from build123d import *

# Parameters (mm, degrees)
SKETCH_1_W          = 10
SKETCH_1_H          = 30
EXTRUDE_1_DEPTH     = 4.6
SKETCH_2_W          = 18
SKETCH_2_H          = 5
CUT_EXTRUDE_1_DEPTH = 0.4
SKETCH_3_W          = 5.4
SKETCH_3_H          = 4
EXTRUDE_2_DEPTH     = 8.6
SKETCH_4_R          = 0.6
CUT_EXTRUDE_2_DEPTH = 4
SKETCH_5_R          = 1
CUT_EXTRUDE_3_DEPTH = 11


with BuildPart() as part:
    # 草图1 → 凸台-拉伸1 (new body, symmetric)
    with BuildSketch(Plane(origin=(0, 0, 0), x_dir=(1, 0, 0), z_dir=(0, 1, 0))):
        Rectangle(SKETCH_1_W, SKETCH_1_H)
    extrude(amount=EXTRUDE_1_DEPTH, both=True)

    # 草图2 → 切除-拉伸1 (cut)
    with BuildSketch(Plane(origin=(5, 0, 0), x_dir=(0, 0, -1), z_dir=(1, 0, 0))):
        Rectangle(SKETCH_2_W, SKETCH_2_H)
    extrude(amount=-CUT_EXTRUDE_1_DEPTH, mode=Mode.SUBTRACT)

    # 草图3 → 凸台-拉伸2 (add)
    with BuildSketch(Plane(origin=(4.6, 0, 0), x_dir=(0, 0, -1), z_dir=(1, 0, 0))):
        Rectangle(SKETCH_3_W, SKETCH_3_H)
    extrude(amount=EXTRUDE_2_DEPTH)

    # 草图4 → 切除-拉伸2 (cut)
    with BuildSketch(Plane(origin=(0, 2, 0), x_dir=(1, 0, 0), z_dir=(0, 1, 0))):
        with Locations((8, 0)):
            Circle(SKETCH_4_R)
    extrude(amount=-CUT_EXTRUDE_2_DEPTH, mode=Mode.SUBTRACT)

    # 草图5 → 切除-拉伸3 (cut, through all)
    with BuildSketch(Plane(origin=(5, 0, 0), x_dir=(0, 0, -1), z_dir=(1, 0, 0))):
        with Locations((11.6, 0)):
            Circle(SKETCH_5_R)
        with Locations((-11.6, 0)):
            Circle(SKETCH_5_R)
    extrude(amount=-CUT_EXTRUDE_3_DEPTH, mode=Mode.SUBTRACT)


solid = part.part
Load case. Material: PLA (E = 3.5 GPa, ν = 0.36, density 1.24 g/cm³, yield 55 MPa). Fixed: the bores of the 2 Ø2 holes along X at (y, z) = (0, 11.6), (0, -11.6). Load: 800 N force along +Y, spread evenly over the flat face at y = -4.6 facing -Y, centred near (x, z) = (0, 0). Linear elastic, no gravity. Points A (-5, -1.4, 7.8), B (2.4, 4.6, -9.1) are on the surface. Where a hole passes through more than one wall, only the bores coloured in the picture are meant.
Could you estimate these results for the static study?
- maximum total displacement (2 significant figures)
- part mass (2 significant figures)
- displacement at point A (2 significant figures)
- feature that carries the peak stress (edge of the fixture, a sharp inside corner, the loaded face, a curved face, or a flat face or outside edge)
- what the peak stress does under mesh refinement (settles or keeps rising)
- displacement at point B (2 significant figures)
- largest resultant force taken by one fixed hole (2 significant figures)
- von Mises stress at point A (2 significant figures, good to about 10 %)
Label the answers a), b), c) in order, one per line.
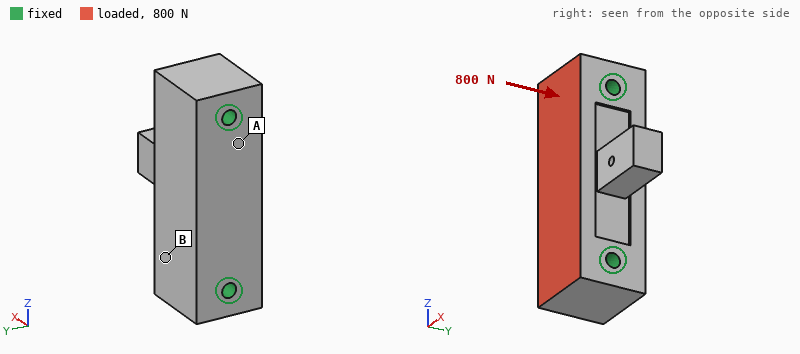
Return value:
a) 51 µm
b) 3.5 g
c) 20 µm
d) edge of the fixture
e) keeps rising
f) 19 µm
g) 400 N
h) 5.9 MPa
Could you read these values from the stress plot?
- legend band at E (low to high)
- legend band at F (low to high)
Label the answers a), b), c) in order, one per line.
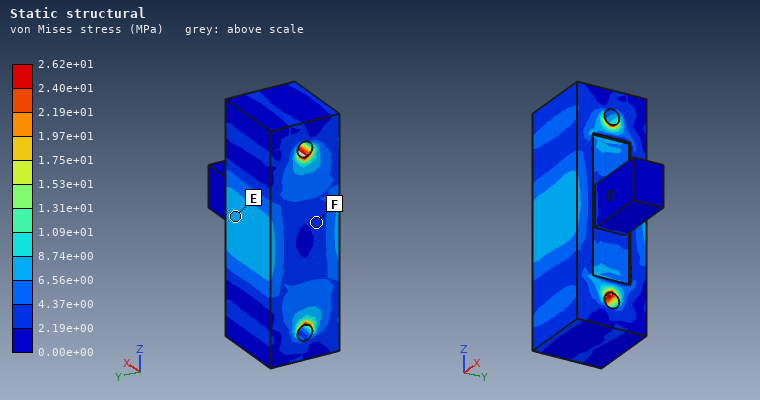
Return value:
a) 6.56e+00 to 8.74e+00 MPa
b) 2.19e+00 to 4.37e+00 MPa
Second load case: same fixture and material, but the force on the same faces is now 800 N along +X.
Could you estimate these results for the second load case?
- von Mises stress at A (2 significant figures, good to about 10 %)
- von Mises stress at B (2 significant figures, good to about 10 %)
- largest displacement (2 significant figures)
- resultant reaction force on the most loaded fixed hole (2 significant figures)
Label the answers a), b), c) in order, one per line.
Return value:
a) 9.3 MPa
b) 3.9 MPa
c) 95 µm
d) 400 N
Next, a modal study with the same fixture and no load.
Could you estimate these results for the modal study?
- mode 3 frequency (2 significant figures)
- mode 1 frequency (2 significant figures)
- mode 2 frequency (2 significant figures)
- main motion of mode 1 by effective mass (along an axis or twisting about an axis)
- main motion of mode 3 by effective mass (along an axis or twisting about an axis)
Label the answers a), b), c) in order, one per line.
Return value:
a) 13 kHz
b) 8500 Hz
c) 12 kHz
d) along Y
e) along Y
